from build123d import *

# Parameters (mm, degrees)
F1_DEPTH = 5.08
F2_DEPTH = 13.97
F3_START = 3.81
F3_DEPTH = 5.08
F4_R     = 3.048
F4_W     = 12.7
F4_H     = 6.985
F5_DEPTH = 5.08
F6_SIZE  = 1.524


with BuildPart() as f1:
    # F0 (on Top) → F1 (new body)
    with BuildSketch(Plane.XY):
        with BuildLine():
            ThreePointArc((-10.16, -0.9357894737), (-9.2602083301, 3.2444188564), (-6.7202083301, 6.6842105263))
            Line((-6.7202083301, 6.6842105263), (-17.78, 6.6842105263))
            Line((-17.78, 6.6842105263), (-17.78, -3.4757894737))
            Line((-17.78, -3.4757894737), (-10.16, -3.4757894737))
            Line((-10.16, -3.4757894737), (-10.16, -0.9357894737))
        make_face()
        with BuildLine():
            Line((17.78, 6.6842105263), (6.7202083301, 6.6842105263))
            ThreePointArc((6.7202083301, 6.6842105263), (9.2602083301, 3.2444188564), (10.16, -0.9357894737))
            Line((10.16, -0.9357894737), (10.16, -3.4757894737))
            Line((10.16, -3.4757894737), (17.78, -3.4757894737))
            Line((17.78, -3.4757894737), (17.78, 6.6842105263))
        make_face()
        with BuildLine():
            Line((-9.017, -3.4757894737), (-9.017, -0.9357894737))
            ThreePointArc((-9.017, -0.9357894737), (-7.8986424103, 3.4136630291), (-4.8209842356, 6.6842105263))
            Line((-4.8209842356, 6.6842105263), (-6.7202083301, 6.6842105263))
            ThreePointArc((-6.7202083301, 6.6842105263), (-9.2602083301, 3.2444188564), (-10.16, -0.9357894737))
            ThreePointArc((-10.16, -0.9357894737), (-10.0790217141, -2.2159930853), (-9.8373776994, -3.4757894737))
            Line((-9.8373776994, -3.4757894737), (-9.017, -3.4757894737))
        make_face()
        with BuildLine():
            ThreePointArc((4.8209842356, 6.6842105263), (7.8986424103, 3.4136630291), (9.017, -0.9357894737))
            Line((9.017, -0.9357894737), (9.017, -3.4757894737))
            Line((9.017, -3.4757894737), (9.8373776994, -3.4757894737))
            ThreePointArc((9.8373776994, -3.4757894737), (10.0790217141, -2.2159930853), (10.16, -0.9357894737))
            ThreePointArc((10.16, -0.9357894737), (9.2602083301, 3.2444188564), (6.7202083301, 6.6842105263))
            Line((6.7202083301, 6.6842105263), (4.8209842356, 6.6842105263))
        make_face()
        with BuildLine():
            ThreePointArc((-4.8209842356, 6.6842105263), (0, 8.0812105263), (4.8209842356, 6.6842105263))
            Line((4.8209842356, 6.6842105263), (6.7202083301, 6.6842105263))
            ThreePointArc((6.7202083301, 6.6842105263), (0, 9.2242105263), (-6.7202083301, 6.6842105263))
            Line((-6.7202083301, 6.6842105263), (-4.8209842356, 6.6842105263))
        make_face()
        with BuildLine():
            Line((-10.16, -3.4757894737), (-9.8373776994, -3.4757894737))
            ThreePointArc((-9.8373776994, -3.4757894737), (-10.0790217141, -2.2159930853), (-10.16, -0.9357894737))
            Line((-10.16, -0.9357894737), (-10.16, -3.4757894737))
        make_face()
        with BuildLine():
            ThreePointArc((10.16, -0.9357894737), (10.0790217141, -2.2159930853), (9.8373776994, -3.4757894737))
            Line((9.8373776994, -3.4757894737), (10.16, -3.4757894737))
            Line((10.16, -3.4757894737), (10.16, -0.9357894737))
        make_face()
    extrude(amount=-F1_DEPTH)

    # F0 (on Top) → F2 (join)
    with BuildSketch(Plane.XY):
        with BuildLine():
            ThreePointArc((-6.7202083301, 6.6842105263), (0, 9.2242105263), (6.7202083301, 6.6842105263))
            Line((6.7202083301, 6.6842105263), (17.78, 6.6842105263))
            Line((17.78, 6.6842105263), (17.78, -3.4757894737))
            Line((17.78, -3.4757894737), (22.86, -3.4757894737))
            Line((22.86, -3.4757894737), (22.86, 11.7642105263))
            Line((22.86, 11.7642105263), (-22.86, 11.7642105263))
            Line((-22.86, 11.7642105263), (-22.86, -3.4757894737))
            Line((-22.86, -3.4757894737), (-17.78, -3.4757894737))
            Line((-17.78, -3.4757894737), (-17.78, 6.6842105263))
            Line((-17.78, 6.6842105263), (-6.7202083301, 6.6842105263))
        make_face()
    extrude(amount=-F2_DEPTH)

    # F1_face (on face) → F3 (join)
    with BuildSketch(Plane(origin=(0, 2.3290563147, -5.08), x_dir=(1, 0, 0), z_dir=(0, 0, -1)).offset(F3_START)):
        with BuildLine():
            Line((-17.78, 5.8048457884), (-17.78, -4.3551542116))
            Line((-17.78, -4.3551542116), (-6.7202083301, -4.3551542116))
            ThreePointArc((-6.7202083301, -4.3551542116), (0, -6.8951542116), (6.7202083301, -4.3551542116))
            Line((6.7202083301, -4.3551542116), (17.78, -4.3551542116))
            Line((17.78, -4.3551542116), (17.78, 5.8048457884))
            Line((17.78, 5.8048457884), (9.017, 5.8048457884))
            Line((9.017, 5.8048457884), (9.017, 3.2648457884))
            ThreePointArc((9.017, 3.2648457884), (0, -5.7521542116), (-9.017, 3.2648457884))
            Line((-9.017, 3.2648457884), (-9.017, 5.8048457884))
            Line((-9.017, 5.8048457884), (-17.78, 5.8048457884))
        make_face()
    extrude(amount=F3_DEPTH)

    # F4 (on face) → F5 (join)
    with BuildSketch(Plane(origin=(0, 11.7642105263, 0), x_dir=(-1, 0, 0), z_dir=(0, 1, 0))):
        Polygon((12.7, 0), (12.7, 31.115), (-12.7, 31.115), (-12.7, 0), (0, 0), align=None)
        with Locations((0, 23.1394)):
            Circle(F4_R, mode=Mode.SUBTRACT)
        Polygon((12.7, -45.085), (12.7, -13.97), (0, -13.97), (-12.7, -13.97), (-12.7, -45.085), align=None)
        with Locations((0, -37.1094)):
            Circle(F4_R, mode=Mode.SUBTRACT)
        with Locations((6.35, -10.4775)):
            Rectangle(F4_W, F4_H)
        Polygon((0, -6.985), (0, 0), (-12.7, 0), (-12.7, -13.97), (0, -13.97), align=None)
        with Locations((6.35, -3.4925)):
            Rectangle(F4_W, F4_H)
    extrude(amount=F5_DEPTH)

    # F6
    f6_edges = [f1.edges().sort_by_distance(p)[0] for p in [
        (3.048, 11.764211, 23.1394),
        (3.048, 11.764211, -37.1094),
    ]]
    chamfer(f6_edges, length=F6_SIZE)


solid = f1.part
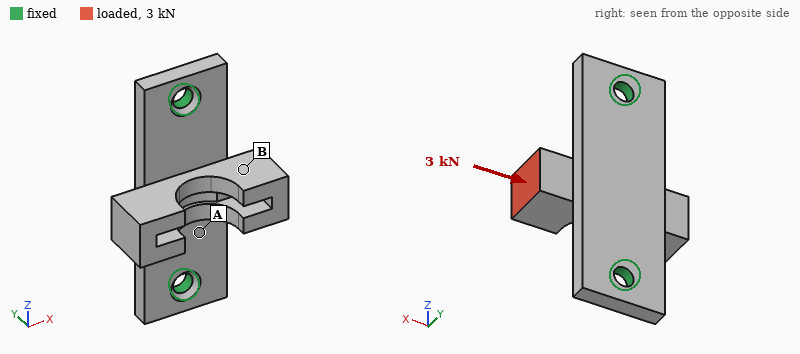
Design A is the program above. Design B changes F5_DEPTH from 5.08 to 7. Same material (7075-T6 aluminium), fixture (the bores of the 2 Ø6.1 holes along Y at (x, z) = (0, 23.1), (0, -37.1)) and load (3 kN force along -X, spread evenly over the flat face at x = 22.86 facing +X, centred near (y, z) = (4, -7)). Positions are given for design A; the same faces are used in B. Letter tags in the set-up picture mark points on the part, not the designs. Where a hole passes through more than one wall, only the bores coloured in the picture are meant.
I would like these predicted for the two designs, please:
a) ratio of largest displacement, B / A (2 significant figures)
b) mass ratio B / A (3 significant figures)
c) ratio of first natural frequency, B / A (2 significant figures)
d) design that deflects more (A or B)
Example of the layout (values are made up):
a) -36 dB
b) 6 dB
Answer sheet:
a) 0.55
b) 1.23
c) 1.4
d) A
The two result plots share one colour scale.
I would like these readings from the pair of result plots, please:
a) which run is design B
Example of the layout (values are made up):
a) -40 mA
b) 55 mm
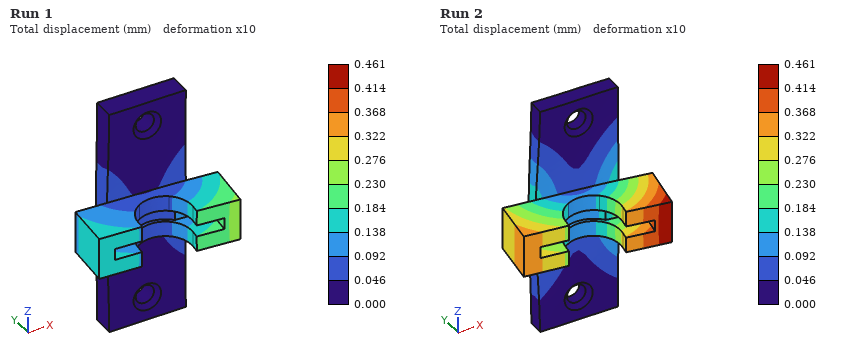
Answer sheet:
a) Run 1
